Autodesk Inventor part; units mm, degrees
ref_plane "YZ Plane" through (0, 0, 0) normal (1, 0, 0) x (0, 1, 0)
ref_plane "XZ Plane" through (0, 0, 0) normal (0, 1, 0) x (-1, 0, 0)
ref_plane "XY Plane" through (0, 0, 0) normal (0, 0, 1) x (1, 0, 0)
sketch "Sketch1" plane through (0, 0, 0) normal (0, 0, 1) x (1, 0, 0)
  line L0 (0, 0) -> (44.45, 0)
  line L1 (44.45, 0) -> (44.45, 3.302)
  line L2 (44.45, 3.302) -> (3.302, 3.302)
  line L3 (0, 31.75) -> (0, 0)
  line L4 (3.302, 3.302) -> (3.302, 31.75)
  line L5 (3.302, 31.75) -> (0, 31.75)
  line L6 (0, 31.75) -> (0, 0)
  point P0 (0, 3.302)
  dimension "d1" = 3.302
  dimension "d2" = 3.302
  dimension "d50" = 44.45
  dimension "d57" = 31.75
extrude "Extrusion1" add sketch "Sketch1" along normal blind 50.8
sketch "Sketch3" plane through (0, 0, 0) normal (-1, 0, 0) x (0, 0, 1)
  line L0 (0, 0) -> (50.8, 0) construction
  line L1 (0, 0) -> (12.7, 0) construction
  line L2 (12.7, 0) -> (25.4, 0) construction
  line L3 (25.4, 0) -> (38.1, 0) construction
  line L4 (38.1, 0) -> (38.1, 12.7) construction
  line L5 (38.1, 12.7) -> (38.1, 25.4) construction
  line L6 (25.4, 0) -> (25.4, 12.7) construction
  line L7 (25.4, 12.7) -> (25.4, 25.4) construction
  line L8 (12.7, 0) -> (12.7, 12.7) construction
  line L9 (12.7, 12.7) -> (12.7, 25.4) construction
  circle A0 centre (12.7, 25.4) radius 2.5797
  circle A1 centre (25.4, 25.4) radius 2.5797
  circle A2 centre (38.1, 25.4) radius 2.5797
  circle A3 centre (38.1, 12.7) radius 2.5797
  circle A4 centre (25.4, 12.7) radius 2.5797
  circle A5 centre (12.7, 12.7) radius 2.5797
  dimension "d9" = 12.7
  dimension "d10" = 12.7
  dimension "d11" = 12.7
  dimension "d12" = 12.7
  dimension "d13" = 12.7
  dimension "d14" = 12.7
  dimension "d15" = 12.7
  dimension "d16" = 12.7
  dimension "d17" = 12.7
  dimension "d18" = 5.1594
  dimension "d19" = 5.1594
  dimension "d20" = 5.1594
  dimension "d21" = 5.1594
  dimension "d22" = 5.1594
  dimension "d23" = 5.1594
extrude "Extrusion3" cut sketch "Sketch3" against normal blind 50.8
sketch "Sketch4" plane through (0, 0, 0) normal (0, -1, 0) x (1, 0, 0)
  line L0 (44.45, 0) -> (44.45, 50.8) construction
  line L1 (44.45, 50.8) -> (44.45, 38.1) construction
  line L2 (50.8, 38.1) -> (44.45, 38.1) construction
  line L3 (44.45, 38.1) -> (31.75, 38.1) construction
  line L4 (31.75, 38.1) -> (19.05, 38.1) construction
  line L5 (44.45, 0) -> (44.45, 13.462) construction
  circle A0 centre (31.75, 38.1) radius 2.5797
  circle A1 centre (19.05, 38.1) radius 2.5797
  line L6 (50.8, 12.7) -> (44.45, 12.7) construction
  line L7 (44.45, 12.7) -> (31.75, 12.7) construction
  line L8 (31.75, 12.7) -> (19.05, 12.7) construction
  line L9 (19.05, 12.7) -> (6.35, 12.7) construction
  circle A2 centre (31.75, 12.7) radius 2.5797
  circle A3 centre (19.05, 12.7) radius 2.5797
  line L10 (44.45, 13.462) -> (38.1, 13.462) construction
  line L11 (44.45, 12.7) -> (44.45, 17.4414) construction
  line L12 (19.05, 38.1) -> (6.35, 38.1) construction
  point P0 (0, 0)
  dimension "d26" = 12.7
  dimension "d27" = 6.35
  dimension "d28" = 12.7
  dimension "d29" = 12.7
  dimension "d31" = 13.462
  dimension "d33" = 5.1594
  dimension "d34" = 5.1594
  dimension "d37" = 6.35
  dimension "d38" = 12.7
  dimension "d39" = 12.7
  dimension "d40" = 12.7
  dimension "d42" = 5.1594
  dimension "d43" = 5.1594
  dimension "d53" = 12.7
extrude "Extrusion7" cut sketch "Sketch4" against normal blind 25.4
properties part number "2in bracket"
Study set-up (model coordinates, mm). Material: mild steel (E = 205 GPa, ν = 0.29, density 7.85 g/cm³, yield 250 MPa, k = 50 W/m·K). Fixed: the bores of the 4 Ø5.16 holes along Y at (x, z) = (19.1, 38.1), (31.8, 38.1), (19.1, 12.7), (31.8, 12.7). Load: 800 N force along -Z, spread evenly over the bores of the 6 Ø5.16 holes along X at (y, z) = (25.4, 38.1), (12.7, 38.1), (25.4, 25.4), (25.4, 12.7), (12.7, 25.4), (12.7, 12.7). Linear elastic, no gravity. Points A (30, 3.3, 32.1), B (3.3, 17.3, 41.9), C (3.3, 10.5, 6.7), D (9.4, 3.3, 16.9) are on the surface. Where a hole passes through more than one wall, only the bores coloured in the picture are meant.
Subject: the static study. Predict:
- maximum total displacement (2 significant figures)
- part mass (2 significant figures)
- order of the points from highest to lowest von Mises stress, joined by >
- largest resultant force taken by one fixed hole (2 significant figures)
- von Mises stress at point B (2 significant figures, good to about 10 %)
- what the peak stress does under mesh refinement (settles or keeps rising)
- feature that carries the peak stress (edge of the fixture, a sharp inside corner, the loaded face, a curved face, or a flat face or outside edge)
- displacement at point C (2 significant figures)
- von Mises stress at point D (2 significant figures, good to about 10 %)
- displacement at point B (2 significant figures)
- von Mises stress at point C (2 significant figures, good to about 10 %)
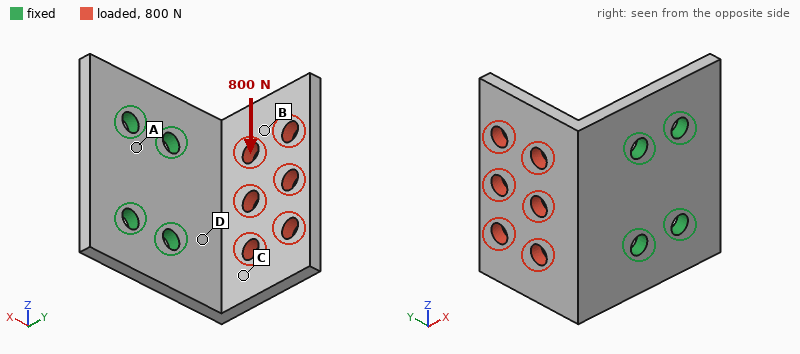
70 µm
91 g
D > C > B > A
740 N
23 MPa
keeps rising
edge of the fixture
33 µm
65 MPa
40 µm
37 MPa
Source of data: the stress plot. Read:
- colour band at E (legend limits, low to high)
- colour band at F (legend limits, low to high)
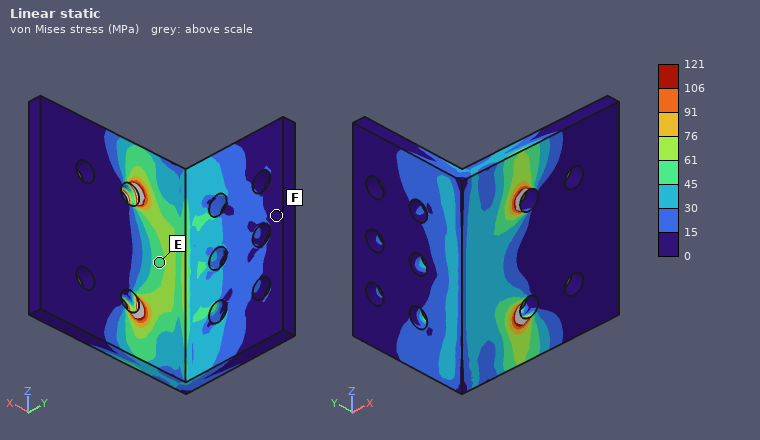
45 to 61 MPa
0 to 15 MPa
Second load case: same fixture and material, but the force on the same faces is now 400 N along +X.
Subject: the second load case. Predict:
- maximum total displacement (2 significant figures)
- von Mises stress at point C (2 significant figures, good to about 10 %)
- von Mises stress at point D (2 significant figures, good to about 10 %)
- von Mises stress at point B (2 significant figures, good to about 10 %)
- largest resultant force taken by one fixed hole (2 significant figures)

0.16 mm
44 MPa
72 MPa
22 MPa
180 N
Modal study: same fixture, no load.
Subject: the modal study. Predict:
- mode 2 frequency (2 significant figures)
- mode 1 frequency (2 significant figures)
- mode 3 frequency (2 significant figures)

3000 Hz
1700 Hz
4800 Hz
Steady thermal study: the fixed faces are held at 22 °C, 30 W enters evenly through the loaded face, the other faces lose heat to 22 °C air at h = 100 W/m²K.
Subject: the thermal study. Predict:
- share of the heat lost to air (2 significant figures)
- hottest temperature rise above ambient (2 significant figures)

61 %
70 K
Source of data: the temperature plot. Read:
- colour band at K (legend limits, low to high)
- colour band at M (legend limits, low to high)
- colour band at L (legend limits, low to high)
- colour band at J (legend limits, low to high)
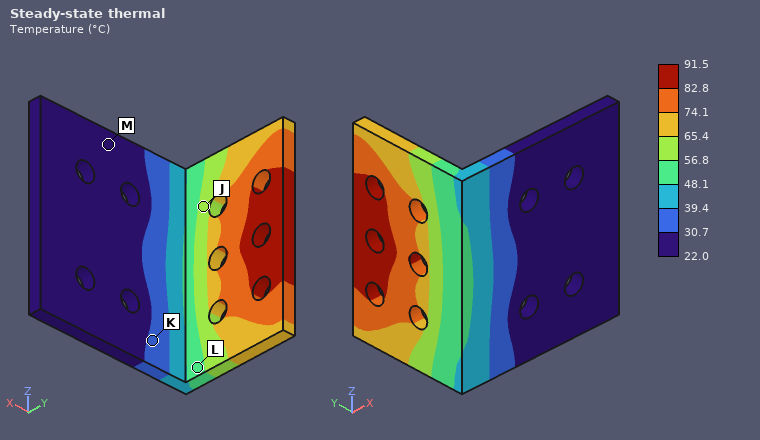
30.7 to 39.4 °C
22.0 to 30.7 °C
48.1 to 56.8 °C
56.8 to 65.4 °C
